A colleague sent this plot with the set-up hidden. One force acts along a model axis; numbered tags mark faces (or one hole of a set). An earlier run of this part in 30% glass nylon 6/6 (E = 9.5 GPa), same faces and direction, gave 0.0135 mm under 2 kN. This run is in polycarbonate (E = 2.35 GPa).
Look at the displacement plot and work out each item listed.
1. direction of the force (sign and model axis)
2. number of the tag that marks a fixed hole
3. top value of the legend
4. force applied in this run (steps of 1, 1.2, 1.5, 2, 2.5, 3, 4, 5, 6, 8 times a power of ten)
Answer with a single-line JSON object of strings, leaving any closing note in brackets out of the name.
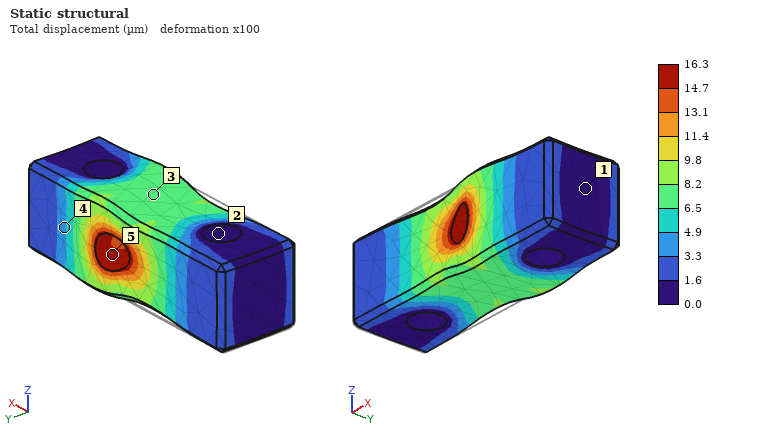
{"direction of the force": "+X", "number of the tag that marks a fixed hole": "2", "top value of the legend": "16.3 µm", "force applied in this run": "600 N"}
